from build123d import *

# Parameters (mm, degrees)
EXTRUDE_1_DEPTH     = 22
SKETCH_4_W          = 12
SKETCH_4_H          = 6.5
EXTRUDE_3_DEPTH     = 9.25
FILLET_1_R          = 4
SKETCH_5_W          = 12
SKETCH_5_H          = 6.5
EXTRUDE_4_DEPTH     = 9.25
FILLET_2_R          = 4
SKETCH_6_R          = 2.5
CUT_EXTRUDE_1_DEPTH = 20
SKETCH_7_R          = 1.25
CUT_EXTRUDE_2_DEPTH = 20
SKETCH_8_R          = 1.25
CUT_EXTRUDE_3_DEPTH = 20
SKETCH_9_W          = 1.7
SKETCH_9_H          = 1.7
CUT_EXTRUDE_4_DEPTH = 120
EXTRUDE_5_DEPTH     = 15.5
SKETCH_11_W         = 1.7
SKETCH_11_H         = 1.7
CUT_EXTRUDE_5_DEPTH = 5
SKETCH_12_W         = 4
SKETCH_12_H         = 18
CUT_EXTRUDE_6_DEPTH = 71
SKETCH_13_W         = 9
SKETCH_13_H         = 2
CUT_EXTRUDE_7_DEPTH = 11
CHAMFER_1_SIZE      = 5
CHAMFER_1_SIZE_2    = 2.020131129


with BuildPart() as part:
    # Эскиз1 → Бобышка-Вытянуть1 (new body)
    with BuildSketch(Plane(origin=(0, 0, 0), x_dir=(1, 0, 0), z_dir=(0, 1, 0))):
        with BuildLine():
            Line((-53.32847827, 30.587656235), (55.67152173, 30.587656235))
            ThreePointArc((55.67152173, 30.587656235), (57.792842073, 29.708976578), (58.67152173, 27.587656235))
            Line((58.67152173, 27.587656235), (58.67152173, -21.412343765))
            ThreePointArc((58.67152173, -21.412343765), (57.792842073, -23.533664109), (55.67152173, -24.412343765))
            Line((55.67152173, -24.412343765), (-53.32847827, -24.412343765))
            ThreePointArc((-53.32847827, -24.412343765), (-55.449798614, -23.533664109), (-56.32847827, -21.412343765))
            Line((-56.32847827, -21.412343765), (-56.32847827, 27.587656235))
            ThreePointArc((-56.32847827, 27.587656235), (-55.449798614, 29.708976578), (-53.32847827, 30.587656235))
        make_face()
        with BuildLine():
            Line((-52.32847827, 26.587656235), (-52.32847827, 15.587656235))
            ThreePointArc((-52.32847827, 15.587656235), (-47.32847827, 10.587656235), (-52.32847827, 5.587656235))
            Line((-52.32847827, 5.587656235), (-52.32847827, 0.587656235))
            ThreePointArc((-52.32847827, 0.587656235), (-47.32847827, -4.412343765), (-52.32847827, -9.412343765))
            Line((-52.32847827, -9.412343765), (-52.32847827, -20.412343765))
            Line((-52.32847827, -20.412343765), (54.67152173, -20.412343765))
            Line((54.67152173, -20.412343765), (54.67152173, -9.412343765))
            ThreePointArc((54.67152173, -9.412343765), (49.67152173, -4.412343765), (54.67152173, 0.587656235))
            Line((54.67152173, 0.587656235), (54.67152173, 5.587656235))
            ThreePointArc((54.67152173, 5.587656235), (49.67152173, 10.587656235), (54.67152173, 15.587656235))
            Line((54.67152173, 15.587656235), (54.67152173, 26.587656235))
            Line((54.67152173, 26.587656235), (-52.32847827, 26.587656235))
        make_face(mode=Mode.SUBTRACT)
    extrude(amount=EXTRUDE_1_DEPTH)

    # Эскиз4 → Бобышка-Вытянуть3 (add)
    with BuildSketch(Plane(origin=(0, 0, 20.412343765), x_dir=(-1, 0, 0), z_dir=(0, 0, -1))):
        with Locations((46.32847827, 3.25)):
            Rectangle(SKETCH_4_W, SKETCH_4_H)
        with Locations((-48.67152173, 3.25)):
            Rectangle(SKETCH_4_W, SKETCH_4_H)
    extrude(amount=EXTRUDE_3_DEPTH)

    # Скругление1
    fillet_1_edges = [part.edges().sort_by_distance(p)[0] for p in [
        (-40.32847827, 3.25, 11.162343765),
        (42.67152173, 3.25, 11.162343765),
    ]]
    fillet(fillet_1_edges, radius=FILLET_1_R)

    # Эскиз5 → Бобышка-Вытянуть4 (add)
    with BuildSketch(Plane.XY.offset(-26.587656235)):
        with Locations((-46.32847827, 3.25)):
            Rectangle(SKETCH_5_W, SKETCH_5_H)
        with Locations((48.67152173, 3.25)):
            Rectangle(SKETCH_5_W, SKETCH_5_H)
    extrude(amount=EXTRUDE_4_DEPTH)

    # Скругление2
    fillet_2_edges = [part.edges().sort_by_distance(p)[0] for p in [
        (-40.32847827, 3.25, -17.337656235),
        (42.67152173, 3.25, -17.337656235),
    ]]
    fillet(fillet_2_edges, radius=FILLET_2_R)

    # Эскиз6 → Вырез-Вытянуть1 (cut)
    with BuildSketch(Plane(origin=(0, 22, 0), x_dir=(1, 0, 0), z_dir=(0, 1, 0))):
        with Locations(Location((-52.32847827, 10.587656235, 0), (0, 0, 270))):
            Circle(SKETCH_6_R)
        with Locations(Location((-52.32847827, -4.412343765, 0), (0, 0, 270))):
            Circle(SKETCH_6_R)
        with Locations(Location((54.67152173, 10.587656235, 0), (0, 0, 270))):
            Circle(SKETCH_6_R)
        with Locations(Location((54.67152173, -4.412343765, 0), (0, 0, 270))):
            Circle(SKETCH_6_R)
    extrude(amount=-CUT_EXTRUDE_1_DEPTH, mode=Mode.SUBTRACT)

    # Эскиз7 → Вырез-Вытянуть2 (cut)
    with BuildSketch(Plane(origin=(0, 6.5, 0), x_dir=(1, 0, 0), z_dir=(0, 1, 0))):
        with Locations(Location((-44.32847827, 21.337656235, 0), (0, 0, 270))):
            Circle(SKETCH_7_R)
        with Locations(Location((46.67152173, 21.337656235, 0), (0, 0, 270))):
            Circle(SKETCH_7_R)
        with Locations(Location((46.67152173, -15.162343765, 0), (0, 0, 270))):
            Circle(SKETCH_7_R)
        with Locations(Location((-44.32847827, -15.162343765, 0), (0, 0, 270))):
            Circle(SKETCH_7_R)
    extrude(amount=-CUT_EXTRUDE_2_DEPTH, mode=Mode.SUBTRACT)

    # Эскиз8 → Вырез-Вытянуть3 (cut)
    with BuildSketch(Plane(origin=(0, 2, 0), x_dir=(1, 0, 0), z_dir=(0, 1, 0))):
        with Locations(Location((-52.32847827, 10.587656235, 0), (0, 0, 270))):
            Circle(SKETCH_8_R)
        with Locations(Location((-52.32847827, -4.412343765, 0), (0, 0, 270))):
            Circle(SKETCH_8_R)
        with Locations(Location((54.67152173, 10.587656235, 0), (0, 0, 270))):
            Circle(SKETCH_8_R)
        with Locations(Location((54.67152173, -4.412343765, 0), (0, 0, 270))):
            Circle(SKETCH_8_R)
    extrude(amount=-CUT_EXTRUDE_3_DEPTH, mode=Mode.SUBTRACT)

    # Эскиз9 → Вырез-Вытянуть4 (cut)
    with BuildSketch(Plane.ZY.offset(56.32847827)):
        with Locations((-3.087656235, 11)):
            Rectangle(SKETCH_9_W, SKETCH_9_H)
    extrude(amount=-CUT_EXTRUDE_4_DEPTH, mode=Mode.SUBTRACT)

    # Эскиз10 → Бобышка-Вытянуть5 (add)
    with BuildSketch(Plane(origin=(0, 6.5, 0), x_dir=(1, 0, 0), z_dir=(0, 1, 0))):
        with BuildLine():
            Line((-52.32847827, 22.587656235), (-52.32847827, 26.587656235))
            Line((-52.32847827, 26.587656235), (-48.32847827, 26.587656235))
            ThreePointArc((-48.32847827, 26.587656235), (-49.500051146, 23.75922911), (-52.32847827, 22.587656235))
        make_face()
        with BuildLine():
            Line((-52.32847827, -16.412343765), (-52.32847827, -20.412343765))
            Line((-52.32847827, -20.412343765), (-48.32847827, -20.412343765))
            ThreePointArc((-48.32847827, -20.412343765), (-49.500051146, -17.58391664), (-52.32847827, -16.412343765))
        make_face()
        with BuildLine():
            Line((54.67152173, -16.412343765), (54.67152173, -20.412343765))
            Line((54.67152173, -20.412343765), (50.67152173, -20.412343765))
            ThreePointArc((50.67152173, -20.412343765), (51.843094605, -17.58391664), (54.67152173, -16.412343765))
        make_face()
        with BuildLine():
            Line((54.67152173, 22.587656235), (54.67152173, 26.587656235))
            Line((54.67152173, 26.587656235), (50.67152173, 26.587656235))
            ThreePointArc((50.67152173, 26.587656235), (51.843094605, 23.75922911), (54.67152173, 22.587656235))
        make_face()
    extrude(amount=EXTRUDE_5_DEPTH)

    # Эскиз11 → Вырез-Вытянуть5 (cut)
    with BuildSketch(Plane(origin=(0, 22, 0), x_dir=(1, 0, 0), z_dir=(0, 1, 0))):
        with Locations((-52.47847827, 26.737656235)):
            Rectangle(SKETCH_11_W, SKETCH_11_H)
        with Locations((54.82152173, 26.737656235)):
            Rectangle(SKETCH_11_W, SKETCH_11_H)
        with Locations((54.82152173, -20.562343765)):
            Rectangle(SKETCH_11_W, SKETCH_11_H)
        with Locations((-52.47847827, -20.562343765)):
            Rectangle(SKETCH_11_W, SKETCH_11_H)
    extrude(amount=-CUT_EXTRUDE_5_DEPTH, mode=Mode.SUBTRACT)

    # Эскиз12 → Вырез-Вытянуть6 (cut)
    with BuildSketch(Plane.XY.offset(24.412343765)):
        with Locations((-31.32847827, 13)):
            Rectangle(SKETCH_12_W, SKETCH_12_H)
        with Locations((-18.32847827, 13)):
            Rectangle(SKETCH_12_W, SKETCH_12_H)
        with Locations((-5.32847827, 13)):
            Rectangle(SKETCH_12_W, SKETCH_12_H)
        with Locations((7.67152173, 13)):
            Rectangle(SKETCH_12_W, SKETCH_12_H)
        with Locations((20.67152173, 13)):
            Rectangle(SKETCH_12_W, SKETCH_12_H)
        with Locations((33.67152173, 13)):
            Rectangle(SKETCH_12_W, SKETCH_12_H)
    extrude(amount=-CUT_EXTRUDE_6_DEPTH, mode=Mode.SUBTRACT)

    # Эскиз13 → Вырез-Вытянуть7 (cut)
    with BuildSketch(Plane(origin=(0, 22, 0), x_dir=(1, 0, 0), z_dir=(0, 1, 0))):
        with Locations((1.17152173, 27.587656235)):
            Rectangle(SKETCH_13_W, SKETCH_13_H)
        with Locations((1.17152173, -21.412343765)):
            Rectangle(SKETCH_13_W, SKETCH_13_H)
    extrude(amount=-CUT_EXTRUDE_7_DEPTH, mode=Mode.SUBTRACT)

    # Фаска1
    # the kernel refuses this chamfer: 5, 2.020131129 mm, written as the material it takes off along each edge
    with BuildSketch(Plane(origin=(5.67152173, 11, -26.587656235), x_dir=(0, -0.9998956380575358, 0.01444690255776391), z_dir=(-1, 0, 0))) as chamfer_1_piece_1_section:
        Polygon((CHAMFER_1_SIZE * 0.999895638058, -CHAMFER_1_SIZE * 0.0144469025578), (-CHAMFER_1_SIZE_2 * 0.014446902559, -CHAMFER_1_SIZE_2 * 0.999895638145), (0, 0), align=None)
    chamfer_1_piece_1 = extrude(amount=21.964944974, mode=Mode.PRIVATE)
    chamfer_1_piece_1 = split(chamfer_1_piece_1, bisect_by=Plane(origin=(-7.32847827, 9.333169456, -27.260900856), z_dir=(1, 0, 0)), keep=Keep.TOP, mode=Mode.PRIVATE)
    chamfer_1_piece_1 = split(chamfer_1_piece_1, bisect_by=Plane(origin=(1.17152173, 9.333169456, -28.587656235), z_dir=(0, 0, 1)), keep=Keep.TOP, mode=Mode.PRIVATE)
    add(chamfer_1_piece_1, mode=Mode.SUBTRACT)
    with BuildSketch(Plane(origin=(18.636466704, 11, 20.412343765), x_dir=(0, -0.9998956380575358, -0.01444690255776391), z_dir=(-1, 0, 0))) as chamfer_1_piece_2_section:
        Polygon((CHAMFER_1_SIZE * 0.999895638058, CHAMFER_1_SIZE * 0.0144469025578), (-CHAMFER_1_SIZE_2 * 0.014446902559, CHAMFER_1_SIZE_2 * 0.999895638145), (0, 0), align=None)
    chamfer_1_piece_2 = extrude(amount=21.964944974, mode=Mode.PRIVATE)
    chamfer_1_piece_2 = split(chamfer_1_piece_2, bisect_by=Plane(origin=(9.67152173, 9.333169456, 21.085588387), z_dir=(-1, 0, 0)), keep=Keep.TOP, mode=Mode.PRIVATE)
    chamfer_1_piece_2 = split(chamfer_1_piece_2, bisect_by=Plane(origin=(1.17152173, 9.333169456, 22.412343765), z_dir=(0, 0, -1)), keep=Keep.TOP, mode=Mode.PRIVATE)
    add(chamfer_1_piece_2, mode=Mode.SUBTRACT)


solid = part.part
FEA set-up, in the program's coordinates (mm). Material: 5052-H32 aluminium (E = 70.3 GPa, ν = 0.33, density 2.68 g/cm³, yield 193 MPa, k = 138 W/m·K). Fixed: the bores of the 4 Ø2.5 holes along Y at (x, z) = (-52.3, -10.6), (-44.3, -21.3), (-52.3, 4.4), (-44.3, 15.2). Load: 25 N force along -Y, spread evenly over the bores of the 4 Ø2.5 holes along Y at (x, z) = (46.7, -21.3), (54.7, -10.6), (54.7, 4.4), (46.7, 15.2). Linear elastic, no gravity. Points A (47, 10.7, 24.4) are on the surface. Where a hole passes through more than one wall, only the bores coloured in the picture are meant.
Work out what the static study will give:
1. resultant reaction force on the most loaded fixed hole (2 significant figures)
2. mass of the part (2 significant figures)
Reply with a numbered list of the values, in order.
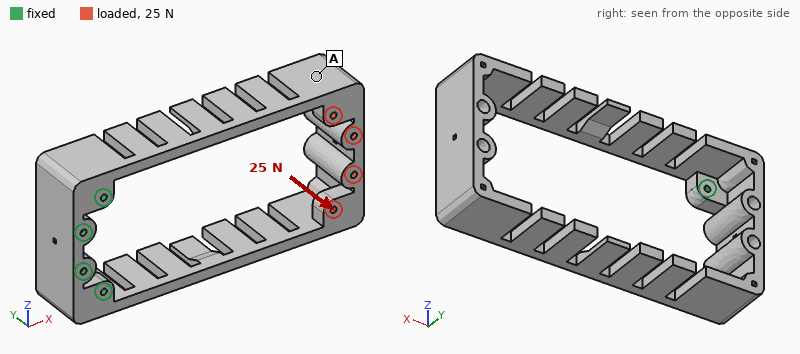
1. 70 N
2. 79 g
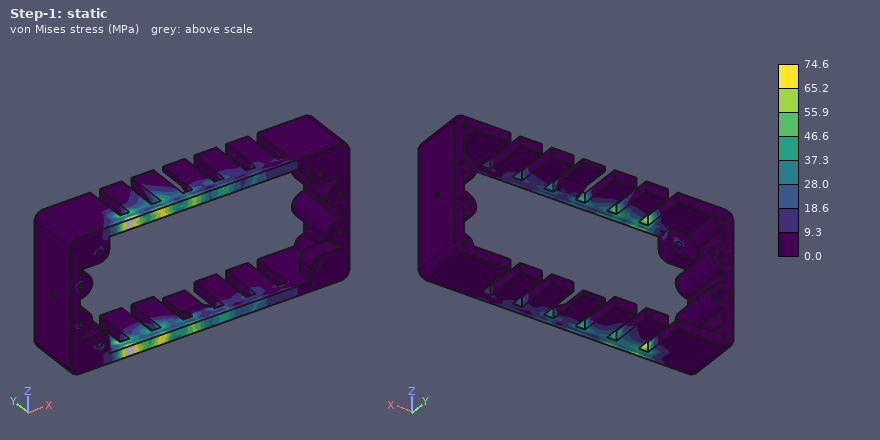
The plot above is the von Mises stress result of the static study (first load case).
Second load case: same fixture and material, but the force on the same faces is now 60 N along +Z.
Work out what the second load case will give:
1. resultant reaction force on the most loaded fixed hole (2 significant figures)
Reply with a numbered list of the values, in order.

1. 170 N
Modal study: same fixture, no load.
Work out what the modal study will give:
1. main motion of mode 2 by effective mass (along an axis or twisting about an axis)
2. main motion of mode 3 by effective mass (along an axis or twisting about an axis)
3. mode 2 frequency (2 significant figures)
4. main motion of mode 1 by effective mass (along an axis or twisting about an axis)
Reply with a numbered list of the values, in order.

1. along Z
2. twisting about X
3. 220 Hz
4. along Y
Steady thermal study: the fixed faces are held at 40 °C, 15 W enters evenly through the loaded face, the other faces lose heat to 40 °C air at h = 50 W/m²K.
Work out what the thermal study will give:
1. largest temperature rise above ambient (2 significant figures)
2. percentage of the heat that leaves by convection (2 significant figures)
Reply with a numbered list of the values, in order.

1. 37 K
2. 94 %
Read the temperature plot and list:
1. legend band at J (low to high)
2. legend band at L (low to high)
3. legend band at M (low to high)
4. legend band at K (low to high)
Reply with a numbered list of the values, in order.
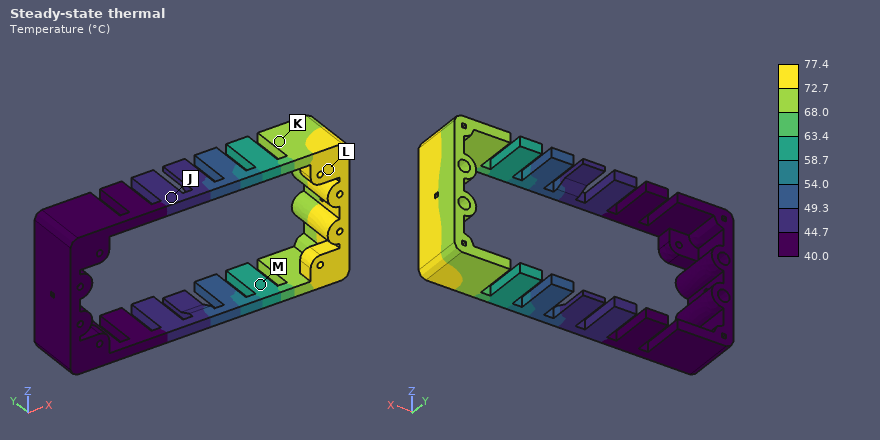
1. 44.7 to 49.3 °C
2. 72.7 to 77.4 °C
3. 58.7 to 63.4 °C
4. 68.0 to 72.7 °C
